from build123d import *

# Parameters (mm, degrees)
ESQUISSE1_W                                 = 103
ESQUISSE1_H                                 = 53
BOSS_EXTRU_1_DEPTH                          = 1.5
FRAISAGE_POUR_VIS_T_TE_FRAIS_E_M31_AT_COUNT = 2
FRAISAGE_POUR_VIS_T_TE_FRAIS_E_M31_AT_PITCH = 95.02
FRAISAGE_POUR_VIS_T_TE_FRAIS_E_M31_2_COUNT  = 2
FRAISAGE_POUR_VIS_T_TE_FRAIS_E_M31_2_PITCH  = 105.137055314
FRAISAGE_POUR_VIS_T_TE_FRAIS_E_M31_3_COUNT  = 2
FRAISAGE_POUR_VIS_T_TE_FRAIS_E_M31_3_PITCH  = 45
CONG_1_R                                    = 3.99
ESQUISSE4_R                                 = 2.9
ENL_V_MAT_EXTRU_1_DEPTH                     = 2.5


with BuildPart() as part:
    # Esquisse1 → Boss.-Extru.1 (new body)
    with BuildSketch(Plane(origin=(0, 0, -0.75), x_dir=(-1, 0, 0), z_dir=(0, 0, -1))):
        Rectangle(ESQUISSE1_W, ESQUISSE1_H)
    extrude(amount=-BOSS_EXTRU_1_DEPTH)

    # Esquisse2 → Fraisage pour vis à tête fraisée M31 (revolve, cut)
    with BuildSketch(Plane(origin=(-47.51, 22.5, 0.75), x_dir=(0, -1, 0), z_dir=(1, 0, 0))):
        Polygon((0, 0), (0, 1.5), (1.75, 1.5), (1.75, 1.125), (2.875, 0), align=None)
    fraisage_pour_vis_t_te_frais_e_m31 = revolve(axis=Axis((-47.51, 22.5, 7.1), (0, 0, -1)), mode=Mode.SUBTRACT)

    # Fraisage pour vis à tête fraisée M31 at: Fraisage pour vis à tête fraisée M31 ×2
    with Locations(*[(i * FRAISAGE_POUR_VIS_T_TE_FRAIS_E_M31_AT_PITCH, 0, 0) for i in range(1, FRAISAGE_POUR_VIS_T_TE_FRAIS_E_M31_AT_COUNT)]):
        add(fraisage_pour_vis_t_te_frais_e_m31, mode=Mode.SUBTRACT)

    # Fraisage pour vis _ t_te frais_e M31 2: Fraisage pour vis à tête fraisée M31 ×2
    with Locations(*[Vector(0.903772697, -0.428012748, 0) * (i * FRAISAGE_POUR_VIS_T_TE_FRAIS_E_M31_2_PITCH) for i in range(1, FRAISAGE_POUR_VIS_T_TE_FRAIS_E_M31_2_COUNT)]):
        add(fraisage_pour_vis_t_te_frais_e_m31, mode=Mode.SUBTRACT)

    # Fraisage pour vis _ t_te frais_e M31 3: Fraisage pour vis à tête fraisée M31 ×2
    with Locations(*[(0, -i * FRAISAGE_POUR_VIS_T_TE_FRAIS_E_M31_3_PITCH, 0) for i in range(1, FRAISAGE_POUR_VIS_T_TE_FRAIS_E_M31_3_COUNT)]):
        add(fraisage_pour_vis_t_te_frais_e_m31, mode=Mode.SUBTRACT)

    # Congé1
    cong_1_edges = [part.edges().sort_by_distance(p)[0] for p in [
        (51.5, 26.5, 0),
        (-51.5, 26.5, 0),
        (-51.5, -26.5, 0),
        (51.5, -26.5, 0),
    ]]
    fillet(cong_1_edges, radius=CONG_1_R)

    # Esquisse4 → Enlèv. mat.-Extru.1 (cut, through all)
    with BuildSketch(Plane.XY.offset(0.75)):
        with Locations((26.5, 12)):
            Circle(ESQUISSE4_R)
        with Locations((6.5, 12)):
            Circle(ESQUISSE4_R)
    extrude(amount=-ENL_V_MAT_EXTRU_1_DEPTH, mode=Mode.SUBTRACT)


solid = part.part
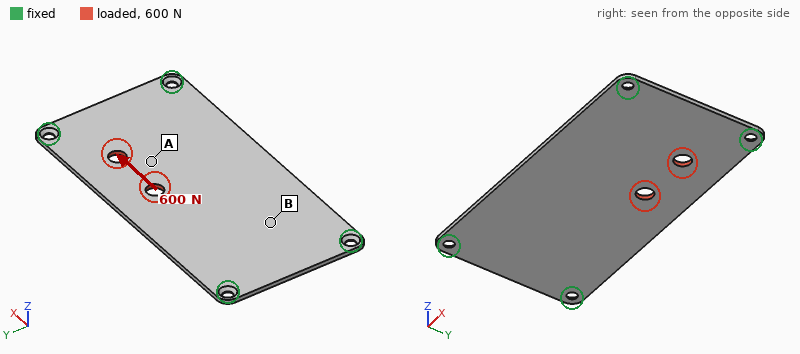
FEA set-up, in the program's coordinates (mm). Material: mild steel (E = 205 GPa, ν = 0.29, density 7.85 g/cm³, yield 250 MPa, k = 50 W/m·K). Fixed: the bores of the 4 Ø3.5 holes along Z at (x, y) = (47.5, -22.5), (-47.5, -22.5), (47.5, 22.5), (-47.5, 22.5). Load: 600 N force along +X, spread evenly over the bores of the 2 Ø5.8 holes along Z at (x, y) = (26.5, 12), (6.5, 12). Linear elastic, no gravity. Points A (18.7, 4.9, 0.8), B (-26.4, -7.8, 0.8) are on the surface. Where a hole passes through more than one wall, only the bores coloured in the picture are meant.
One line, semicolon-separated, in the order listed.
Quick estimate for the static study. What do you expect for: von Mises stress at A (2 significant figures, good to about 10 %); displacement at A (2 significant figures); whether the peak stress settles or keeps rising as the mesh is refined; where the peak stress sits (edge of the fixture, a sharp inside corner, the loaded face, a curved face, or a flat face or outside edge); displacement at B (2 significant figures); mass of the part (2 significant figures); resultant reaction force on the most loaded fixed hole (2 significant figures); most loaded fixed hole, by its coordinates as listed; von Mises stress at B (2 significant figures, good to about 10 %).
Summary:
6.3 MPa; 3.8 µm; keeps rising; edge of the fixture; 1.6 µm; 63 g; 230 N; (47.5, 22.5); 2.8 MPa
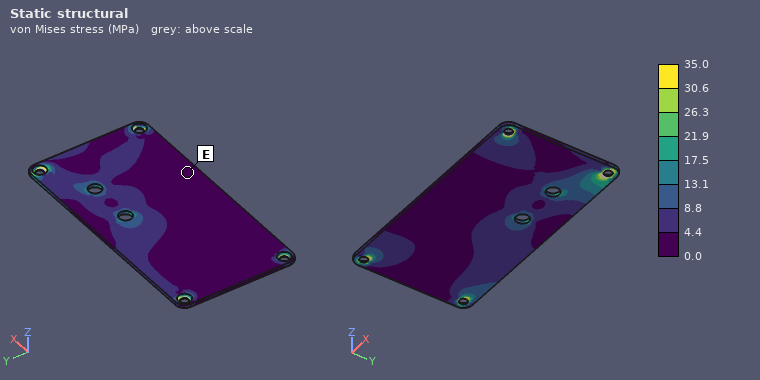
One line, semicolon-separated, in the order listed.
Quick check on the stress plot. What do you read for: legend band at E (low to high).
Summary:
0.0 to 4.4 MPa
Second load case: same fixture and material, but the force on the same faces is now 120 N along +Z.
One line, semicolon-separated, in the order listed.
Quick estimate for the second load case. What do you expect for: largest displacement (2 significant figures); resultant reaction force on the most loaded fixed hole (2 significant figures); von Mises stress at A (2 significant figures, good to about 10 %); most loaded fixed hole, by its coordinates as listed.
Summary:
0.26 mm; 190 N; 42 MPa; (47.5, 22.5)
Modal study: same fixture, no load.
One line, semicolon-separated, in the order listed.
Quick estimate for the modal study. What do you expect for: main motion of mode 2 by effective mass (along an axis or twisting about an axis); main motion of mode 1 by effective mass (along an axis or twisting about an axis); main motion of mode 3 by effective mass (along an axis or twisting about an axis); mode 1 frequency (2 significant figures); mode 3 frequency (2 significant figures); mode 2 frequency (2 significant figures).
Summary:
twisting about X; along Z; twisting about Y; 690 Hz; 1900 Hz; 1300 Hz
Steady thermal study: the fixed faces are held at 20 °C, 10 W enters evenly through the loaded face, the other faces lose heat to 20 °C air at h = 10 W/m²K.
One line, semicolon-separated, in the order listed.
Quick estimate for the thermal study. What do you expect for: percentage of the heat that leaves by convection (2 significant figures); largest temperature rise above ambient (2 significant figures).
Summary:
31 %; 67 K
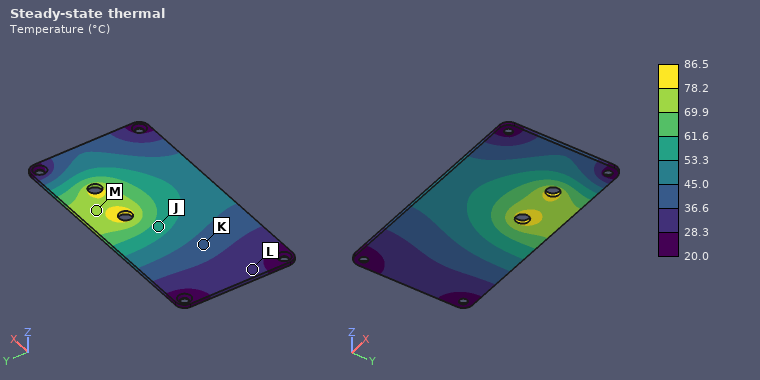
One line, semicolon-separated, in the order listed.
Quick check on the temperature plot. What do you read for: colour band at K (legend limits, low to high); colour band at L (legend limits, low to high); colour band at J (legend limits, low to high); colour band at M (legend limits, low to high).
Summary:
36.6 to 45.0 °C; 28.3 to 36.6 °C; 53.3 to 61.6 °C; 69.9 to 78.2 °C
